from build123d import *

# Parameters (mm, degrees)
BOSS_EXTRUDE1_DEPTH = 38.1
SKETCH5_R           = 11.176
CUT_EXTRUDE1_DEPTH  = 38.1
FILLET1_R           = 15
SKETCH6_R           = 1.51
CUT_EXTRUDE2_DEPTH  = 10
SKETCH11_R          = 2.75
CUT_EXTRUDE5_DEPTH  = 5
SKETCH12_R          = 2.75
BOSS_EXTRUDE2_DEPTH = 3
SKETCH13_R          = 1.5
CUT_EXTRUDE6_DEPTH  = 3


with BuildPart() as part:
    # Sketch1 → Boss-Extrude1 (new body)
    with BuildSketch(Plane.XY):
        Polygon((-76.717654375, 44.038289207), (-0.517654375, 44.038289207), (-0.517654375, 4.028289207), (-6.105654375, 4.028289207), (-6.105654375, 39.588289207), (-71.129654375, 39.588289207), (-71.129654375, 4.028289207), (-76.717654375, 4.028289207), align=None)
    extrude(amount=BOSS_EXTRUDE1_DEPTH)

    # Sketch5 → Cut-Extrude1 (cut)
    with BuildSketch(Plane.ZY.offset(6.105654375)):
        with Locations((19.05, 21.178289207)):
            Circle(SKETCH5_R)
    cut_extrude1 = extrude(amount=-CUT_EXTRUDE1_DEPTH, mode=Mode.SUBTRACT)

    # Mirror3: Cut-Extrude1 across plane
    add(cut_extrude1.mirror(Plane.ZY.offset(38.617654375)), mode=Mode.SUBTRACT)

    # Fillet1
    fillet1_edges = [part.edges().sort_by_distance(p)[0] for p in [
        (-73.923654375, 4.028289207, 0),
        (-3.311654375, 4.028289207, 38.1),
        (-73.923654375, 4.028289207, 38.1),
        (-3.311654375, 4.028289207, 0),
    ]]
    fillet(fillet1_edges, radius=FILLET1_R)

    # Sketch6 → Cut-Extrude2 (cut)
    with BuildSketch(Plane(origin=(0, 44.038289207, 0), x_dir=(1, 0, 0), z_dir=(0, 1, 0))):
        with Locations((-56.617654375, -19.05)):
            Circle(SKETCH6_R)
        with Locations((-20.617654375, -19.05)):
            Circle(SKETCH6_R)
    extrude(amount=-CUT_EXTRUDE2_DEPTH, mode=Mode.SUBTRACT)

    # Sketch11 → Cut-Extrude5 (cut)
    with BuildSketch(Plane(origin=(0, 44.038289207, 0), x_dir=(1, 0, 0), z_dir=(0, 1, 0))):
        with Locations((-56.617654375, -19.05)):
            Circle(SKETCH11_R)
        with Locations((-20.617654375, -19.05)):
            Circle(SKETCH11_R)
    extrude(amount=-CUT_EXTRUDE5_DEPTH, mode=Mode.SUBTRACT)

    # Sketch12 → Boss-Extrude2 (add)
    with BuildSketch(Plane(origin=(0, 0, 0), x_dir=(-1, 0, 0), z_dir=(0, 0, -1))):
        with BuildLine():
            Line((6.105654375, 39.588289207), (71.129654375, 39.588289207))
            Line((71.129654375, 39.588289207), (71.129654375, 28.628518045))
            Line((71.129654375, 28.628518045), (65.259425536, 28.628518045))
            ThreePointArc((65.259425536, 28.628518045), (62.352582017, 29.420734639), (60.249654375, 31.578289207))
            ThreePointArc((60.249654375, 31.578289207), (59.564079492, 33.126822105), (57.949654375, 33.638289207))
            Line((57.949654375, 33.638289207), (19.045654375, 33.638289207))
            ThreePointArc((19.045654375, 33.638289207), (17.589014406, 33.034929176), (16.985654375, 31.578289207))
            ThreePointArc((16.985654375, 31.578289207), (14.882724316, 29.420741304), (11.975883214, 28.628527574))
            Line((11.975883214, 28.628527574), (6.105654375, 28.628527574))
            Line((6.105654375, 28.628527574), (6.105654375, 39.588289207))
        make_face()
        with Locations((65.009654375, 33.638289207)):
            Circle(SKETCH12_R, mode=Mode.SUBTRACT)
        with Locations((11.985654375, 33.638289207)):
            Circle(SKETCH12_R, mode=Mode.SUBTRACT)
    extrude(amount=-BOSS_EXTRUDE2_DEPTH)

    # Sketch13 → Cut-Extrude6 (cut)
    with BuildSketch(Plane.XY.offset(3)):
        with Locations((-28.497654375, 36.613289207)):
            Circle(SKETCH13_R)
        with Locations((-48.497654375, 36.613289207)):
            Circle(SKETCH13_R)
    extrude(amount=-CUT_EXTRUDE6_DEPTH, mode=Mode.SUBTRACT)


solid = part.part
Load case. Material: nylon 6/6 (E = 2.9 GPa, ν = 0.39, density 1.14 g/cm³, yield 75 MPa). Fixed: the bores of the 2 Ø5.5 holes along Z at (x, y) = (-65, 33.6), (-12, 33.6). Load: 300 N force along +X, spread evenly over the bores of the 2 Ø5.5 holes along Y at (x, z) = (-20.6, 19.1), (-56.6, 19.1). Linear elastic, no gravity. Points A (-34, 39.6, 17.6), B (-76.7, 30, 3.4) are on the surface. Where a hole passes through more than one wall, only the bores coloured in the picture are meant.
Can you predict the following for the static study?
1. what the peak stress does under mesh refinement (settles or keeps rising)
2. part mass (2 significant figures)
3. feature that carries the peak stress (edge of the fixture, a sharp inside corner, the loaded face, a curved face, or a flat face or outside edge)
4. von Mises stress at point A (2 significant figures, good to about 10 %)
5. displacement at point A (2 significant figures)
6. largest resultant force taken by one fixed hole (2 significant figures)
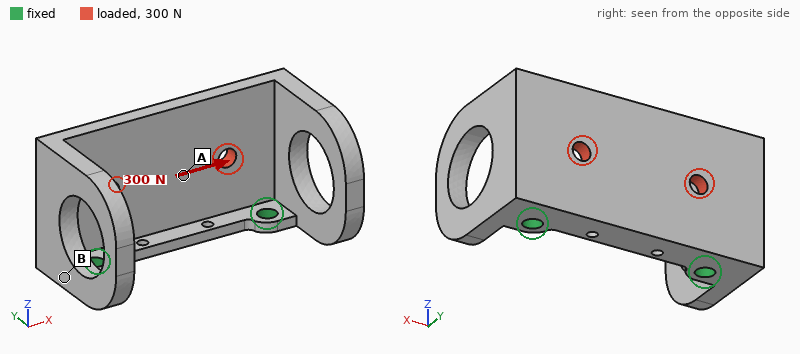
keeps rising
27 g
edge of the fixture
2.4 MPa
0.074 mm
180 N
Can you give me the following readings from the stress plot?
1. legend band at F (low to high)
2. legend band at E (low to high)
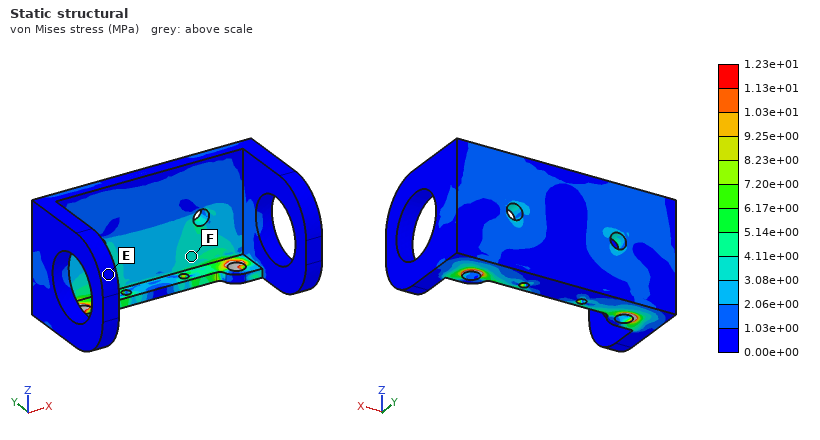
3.08e+00 to 4.11e+00 MPa
0.00e+00 to 1.03e+00 MPa
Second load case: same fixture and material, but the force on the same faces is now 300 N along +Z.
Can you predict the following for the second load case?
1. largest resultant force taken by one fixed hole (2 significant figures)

150 N
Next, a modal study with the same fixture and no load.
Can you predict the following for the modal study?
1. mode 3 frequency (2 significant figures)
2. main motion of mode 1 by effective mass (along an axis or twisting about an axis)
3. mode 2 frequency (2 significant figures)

880 Hz
along Y
630 Hz
